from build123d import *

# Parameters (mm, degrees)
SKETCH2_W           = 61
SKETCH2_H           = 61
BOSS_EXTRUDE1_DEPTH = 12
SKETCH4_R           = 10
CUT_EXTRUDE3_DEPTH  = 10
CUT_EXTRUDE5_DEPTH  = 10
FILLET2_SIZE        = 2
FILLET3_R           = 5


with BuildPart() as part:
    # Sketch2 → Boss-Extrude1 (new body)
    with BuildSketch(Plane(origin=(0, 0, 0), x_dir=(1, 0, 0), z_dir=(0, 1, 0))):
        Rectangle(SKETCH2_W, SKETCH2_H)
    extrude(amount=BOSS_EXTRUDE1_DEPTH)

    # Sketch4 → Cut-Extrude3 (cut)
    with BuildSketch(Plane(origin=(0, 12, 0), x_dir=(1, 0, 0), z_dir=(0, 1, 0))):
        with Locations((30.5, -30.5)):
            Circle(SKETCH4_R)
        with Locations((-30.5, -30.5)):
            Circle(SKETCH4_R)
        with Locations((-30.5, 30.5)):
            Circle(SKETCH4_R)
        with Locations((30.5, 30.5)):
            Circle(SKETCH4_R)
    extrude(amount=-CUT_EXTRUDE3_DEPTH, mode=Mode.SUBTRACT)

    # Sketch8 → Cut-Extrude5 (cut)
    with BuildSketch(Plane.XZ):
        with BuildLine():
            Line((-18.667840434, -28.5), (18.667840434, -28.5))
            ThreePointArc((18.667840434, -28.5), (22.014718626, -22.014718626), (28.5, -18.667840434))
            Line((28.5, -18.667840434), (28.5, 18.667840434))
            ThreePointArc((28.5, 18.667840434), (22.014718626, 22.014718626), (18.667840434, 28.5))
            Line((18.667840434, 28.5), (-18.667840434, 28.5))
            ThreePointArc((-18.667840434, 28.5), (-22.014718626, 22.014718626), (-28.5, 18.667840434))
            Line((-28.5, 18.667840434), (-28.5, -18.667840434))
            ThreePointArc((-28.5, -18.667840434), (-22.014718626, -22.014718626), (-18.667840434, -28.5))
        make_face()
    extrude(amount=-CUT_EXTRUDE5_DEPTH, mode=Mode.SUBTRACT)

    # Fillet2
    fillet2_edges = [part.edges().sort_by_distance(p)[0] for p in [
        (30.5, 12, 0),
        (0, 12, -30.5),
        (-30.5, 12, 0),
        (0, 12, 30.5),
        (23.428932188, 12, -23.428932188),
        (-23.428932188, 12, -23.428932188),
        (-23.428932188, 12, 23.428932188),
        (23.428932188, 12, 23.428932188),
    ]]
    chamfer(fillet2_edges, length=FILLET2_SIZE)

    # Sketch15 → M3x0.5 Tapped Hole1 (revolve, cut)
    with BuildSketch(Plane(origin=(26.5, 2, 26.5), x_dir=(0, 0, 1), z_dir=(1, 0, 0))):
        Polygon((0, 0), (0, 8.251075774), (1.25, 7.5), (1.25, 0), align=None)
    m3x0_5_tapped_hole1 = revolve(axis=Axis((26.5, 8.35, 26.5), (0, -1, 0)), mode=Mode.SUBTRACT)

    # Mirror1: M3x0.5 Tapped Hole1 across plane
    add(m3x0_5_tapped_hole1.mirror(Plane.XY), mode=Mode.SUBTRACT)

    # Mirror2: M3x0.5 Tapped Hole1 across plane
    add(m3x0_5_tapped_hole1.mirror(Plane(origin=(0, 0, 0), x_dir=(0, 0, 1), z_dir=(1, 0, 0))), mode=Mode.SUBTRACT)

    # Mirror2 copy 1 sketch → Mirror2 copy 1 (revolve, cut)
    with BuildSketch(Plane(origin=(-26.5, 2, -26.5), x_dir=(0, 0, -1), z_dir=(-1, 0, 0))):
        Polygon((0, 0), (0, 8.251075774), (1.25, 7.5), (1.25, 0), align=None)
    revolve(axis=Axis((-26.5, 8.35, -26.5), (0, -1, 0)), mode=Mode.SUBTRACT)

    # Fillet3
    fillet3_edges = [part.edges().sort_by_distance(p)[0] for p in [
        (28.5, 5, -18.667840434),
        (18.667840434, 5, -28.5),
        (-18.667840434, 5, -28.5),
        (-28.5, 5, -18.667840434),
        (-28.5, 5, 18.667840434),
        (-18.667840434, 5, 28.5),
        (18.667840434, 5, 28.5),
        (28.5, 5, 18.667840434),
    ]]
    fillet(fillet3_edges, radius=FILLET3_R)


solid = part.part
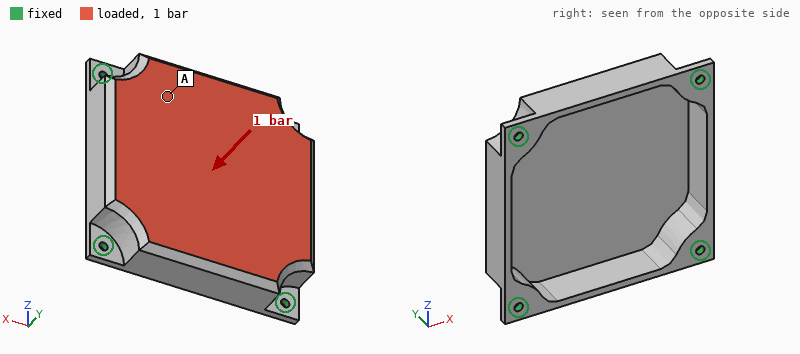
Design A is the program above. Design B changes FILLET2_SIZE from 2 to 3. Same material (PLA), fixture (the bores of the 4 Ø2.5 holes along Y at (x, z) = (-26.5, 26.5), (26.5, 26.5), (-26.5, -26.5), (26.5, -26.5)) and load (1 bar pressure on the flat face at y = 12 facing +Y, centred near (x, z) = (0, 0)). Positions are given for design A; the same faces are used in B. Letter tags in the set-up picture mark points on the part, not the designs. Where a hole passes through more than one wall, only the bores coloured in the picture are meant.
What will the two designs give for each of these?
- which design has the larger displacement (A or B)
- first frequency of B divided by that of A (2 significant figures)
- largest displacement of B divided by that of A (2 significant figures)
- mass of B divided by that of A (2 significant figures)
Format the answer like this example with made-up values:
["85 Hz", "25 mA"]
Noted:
["B", "0.92", "1.2", "0.95"]
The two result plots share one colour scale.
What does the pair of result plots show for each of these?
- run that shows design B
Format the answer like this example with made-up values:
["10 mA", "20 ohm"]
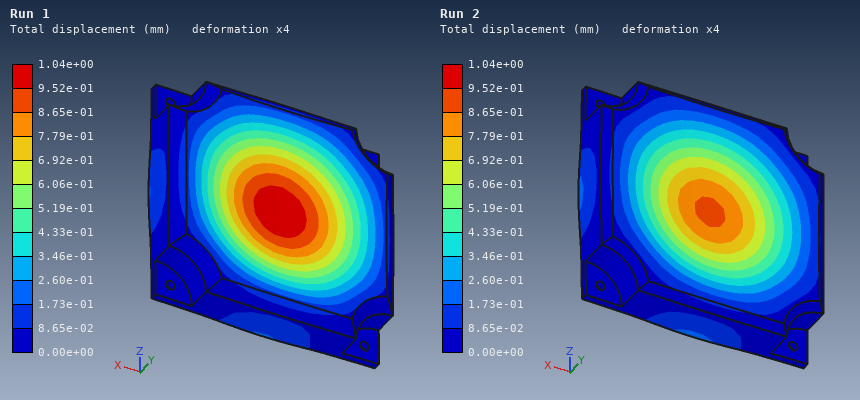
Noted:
["Run 1"]
